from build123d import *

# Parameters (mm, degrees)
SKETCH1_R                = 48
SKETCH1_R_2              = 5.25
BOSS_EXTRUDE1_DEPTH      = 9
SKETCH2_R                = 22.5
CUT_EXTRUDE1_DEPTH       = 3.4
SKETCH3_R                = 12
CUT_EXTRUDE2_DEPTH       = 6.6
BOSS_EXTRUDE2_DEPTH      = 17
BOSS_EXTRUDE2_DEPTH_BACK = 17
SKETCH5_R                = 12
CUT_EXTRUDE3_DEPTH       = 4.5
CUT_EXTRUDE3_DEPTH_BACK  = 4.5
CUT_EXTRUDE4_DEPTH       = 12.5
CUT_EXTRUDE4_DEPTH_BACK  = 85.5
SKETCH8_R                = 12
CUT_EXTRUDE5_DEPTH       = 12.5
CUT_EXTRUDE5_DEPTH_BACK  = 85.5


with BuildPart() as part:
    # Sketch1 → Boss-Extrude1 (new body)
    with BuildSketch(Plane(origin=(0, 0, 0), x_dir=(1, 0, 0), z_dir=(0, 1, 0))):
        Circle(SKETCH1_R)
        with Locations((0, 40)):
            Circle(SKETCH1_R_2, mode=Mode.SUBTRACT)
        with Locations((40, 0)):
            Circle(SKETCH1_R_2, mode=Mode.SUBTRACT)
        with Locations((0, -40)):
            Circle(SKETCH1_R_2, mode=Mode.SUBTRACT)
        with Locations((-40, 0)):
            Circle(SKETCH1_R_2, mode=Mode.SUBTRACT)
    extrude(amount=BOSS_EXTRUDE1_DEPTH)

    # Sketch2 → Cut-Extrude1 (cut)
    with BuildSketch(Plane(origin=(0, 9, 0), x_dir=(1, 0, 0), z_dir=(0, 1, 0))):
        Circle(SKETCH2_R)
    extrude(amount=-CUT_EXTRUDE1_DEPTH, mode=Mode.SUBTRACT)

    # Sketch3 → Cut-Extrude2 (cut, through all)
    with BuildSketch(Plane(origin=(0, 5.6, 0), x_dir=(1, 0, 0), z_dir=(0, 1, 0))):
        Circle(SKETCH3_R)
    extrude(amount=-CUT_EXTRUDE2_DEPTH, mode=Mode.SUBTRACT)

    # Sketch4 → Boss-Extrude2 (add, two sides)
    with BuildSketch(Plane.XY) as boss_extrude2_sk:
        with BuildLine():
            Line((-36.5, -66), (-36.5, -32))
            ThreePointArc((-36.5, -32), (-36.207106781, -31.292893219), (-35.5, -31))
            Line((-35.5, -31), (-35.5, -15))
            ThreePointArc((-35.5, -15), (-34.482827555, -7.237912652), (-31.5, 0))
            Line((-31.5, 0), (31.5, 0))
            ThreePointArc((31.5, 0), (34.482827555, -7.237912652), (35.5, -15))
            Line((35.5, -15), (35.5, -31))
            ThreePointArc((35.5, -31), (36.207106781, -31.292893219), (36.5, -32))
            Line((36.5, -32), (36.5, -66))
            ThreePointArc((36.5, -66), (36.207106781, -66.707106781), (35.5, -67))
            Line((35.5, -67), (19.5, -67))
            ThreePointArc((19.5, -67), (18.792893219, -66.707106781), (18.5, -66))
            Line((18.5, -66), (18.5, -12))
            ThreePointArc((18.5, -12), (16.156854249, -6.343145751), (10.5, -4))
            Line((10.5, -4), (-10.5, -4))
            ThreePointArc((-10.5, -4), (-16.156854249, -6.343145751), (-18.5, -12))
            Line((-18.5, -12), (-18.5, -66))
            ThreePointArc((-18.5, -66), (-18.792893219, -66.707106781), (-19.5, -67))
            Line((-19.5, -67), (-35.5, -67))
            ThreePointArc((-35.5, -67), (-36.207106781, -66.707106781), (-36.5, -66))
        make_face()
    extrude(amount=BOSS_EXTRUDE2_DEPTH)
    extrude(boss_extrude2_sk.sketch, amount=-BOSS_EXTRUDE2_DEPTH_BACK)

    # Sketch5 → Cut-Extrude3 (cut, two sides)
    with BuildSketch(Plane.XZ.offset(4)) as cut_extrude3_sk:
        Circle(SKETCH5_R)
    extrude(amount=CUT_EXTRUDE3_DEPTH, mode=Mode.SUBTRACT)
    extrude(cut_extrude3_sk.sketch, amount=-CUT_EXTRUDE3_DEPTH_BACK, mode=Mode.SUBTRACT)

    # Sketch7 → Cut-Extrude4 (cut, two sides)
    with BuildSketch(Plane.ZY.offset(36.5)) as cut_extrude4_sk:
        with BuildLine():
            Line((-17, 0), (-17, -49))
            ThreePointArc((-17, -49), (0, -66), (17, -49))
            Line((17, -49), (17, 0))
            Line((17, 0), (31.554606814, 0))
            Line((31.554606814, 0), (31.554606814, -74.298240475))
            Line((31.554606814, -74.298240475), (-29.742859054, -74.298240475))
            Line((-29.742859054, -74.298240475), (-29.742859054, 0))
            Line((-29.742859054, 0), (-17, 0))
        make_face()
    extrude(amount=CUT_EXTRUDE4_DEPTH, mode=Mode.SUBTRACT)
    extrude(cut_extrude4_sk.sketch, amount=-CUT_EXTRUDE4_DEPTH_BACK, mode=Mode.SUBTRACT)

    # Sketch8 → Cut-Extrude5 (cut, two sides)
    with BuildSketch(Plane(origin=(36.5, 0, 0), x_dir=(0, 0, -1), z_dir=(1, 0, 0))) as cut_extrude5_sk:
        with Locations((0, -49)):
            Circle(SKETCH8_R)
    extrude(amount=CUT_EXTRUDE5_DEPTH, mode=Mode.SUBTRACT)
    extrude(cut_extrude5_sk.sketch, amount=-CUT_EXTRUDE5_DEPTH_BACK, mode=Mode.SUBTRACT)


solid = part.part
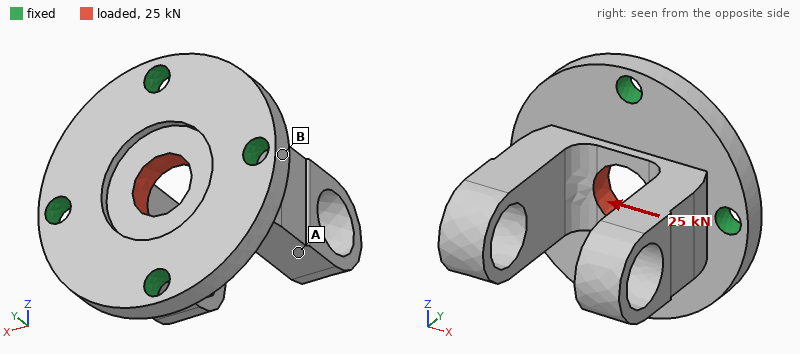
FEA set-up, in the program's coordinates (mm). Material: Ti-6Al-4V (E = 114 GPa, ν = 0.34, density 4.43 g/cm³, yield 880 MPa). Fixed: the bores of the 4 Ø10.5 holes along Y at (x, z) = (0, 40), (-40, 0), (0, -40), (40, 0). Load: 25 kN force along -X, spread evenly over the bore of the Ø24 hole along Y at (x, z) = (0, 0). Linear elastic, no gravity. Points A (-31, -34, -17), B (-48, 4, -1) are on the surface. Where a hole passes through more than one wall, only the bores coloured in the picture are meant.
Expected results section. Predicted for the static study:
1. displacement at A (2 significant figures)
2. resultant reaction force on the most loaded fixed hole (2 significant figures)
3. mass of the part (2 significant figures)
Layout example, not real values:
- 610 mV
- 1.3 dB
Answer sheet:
- 14 µm
- 8.4 kN
- 510 g
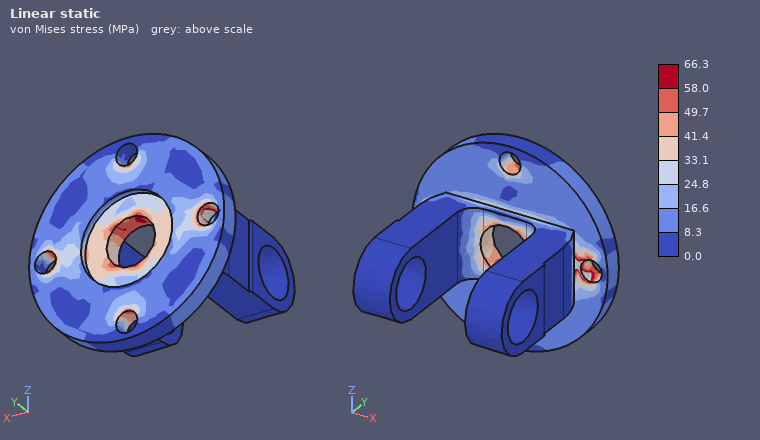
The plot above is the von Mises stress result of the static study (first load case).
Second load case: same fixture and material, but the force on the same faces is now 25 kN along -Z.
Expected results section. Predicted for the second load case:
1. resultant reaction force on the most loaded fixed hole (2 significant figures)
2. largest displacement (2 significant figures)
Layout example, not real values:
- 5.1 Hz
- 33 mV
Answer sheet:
- 7.9 kN
- 18 µm
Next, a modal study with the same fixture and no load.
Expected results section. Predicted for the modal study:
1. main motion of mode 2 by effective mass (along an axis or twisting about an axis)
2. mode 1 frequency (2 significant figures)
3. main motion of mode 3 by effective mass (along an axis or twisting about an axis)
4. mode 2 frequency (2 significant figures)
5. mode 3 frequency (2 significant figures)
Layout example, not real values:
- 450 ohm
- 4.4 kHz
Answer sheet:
- along X
- 2800 Hz
- along Z
- 3200 Hz
- 3800 Hz
